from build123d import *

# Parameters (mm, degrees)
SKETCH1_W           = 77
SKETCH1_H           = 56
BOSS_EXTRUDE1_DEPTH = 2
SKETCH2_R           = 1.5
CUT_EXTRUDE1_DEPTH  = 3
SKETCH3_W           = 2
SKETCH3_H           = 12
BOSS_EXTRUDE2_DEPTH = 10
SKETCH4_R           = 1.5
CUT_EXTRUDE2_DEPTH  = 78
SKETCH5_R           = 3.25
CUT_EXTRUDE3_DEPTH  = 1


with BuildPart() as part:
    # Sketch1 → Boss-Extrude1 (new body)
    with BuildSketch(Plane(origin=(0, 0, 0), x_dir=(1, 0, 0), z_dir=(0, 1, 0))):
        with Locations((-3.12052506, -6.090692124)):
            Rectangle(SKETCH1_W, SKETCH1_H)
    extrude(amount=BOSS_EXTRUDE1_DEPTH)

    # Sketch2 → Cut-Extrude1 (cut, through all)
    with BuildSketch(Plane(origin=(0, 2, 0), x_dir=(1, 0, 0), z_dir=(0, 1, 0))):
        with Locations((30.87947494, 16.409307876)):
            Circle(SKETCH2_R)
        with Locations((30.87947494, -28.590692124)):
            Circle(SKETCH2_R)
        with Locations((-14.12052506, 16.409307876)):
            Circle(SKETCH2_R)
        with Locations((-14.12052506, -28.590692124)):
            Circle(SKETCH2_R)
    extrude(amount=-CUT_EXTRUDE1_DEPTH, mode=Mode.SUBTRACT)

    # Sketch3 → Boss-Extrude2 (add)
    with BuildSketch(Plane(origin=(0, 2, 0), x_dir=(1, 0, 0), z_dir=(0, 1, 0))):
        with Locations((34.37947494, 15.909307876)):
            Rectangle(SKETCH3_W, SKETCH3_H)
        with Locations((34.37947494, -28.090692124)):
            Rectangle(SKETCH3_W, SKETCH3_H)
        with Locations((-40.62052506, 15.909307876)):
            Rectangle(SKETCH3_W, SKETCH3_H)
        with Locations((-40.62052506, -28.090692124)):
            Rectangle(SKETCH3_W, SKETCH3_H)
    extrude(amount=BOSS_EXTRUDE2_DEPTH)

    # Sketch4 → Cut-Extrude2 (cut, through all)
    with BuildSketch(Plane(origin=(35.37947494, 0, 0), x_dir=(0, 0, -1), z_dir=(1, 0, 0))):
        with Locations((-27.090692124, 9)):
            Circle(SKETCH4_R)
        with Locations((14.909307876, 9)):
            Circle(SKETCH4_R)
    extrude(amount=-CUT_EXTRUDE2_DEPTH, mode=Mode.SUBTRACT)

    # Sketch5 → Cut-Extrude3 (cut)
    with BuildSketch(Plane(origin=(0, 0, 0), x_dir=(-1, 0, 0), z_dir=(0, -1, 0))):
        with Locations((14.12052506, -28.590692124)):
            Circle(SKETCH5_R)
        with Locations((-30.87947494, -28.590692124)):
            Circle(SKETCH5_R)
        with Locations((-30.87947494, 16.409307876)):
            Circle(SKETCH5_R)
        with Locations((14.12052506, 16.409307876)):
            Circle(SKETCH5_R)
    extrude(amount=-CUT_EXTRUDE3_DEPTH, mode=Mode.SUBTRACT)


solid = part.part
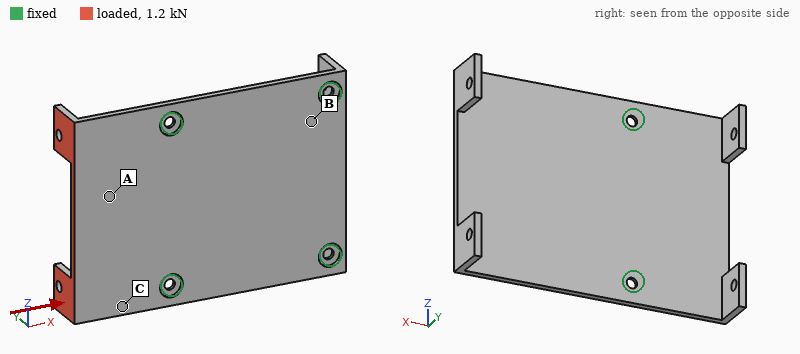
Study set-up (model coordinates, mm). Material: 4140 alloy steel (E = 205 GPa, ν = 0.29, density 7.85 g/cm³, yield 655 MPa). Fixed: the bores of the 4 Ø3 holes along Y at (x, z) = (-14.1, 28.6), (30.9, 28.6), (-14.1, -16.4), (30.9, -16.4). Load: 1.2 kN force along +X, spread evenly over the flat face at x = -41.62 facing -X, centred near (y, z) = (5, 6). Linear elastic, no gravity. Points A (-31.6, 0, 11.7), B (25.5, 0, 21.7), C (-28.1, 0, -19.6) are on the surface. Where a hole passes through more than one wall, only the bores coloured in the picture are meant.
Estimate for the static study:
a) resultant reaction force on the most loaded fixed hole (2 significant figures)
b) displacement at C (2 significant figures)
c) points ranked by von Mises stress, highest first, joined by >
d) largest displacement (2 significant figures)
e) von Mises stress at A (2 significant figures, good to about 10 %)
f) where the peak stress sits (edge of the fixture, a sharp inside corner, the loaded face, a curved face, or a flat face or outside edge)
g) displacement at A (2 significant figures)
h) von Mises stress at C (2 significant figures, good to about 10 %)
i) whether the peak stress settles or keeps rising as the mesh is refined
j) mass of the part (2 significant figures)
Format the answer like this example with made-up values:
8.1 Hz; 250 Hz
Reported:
730 N; 0.092 mm; C > A > B; 0.44 mm; 89 MPa; edge of the fixture; 0.17 mm; 140 MPa; keeps rising; 74 g
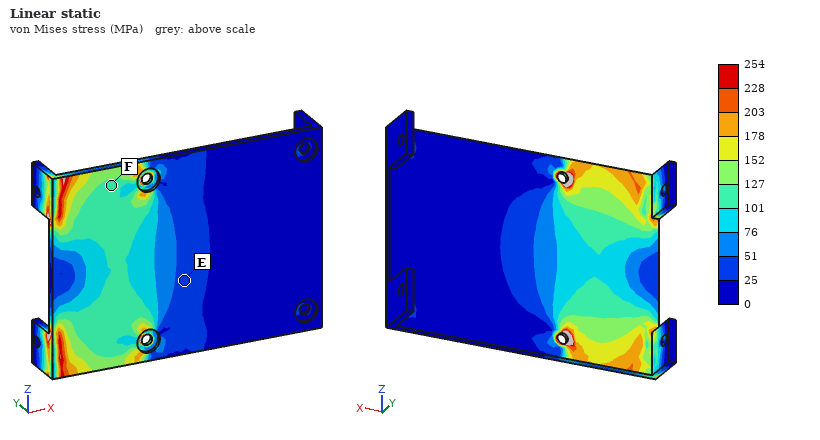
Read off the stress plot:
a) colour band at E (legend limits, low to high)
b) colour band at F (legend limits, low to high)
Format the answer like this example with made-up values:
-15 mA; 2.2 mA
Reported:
25 to 51 MPa; 101 to 127 MPa
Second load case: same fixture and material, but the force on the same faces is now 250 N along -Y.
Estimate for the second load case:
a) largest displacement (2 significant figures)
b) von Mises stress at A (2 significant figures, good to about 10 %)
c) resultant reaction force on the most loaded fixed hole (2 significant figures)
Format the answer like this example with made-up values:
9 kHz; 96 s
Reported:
0.43 mm; 68 MPa; 470 N
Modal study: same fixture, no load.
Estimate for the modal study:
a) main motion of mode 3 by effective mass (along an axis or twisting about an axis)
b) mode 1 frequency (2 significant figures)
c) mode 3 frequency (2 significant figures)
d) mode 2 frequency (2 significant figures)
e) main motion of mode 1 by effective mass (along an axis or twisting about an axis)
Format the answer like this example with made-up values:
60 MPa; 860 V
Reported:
along Y; 1300 Hz; 3000 Hz; 2100 Hz; along Y
